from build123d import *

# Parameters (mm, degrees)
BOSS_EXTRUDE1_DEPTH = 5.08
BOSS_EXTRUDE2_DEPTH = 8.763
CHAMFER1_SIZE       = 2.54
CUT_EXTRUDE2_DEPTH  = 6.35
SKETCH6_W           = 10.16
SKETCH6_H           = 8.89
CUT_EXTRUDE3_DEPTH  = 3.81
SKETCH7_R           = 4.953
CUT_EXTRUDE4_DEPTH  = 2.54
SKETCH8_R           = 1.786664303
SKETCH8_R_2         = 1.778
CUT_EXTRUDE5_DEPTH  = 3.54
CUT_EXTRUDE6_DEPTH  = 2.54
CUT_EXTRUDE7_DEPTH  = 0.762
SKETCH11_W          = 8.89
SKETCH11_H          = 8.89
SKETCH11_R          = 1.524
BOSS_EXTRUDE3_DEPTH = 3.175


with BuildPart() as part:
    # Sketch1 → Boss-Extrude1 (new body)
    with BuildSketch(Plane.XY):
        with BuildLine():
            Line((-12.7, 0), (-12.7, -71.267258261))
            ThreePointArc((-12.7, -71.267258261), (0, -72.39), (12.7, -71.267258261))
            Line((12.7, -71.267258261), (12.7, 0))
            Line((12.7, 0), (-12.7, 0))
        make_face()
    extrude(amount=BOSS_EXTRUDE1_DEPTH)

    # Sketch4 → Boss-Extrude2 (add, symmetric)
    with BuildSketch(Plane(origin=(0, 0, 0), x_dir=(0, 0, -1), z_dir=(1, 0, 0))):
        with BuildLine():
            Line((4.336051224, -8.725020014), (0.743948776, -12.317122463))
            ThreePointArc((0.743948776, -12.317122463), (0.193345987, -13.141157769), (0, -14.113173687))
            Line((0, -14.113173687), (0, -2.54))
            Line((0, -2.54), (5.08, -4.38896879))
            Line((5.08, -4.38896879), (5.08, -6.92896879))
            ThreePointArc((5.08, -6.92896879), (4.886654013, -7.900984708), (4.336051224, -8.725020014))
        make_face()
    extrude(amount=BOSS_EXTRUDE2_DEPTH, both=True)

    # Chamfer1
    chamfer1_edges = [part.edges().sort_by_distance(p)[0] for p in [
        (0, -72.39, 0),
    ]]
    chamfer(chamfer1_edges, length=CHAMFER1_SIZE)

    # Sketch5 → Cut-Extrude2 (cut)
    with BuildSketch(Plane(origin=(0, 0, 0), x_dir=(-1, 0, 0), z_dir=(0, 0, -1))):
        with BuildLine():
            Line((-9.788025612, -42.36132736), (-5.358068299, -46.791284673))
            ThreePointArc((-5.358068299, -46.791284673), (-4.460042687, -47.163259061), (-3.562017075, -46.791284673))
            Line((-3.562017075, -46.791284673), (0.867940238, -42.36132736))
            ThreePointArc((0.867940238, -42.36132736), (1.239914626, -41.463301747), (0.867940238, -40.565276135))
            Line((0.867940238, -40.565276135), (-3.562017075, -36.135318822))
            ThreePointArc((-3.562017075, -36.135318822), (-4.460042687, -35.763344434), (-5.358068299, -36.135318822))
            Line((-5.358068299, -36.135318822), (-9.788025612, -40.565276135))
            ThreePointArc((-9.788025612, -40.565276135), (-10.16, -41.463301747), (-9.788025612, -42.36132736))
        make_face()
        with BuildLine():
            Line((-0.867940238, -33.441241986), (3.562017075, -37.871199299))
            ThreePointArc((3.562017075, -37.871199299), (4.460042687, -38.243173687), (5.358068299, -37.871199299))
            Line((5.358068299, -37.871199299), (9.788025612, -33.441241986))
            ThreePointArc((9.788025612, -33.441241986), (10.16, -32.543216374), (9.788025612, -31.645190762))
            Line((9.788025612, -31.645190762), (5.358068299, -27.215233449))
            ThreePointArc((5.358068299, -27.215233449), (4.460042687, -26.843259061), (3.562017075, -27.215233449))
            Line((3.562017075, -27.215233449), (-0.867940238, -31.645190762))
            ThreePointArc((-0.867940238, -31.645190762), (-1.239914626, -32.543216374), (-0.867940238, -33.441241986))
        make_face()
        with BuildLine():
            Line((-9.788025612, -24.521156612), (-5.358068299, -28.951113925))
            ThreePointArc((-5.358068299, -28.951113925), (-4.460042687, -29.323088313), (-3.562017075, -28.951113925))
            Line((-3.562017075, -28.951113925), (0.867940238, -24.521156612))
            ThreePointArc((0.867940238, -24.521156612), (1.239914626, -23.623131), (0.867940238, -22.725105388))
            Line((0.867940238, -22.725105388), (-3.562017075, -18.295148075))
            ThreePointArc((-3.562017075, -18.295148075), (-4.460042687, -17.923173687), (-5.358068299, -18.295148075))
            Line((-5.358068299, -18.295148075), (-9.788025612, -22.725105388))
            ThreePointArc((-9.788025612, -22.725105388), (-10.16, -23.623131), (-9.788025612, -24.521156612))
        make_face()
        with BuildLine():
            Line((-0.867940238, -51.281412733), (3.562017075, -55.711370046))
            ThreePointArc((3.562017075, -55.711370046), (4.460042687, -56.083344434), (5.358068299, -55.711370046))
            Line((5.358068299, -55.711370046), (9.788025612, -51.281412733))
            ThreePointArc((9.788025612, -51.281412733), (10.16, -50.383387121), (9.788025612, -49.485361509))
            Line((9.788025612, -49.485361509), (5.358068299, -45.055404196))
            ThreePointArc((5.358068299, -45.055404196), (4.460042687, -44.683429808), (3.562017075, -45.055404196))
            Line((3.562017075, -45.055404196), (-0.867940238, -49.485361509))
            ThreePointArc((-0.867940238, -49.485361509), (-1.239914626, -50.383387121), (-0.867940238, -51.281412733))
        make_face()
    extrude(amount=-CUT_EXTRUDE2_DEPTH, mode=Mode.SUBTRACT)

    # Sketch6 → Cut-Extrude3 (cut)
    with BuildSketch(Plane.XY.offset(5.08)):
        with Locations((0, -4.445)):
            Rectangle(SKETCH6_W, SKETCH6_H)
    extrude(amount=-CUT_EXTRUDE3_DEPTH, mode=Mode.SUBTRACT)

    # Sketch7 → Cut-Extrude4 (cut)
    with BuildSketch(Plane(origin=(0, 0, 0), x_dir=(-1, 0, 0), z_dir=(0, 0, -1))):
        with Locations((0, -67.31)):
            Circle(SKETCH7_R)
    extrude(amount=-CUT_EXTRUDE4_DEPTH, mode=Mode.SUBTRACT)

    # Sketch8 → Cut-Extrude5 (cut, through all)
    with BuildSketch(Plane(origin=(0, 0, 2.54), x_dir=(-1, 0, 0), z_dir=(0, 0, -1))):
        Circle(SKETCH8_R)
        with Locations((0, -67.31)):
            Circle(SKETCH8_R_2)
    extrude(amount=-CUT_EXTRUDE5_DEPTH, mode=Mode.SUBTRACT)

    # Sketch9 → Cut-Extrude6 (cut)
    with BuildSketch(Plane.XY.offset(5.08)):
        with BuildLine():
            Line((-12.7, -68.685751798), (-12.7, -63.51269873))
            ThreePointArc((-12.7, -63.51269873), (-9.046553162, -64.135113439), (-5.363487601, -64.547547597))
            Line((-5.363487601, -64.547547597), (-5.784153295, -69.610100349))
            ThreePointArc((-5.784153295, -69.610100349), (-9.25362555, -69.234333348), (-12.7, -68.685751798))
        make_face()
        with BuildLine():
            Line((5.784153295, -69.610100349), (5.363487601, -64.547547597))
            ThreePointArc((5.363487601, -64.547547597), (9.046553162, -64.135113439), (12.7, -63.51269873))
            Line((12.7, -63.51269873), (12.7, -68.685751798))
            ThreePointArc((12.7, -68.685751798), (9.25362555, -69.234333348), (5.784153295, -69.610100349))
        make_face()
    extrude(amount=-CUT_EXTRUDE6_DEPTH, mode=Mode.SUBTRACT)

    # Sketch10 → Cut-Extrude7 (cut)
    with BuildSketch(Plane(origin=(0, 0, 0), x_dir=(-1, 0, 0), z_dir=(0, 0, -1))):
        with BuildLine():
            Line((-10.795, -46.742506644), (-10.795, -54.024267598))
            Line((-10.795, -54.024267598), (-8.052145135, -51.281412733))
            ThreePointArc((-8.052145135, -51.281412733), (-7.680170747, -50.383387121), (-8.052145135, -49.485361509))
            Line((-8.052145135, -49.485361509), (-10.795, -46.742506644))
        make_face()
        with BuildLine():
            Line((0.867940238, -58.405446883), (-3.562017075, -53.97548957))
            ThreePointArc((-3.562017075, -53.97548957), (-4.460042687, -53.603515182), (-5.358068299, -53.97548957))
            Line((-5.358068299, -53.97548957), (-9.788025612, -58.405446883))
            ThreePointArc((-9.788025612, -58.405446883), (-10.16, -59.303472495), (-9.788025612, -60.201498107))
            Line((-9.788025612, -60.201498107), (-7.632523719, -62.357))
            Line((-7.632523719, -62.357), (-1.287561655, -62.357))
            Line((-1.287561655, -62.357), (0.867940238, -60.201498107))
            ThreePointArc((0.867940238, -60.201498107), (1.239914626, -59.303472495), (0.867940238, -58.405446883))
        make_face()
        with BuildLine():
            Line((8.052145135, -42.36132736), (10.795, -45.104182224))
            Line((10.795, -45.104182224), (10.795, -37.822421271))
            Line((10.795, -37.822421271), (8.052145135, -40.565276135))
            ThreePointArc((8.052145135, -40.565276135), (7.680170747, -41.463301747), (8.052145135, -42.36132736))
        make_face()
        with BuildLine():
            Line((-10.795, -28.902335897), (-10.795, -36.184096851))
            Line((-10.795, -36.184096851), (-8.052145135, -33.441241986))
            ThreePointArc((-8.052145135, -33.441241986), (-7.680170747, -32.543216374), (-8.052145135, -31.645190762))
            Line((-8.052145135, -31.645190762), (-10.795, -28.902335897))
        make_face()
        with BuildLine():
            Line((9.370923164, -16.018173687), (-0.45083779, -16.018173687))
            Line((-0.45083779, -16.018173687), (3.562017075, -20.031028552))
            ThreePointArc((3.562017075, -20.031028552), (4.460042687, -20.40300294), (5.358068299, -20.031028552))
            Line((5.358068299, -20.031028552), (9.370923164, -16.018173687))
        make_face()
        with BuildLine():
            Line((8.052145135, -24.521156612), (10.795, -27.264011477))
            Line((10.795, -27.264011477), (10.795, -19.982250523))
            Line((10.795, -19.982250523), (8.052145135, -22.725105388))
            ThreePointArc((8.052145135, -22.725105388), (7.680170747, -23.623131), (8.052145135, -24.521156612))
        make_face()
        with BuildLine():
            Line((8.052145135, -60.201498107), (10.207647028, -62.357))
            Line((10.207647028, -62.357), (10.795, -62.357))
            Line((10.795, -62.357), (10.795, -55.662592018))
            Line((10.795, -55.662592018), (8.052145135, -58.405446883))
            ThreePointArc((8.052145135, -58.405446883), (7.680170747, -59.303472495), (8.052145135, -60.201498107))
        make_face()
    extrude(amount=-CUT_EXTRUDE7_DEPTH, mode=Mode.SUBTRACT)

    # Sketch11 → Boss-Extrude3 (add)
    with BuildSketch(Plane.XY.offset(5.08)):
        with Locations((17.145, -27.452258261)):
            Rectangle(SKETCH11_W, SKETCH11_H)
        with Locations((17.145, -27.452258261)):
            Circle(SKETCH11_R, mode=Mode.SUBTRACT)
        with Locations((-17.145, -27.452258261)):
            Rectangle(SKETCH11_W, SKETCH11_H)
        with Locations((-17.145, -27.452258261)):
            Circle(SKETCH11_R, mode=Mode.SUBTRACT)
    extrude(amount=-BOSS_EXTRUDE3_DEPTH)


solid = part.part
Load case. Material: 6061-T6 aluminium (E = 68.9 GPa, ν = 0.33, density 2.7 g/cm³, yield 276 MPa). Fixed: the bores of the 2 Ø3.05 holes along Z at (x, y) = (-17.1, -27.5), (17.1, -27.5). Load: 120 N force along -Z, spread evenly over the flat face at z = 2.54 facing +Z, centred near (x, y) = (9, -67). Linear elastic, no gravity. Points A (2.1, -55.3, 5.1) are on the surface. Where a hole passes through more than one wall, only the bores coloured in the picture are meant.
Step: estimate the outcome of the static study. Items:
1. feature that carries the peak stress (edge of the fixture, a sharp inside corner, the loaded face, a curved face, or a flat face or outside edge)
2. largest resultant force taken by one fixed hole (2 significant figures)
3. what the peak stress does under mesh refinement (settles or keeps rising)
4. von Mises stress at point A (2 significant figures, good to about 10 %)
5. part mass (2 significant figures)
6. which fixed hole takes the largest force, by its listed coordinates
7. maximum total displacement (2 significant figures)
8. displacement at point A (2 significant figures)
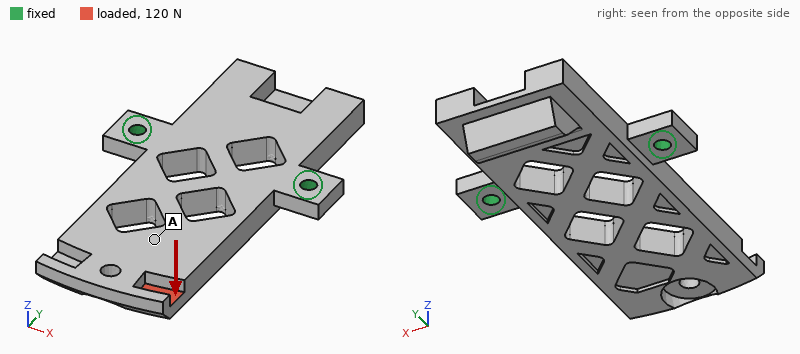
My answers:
edge of the fixture
120 N
keeps rising
23 MPa
21 g
(17.1, -27.5)
0.58 mm
0.30 mm
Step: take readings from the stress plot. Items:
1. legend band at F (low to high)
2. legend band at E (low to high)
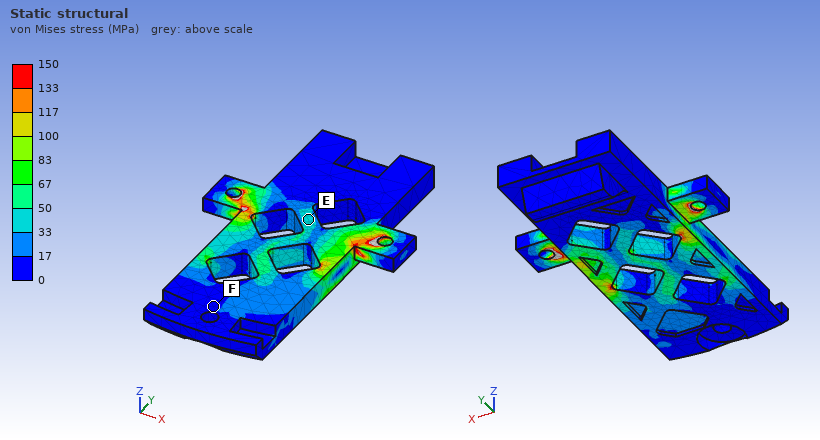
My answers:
0 to 17 MPa
33 to 50 MPa
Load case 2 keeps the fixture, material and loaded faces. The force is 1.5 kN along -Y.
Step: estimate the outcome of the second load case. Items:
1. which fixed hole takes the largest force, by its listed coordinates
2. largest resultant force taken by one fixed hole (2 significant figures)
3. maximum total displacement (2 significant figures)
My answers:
(17.1, -27.5)
1.2 kN
0.10 mm
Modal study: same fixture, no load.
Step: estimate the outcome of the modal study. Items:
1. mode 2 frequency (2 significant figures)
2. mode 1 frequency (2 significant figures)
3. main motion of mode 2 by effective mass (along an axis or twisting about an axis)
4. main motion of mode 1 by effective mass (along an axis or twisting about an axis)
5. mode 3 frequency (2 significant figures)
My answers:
2800 Hz
1200 Hz
along Z
along Z
5700 Hz
